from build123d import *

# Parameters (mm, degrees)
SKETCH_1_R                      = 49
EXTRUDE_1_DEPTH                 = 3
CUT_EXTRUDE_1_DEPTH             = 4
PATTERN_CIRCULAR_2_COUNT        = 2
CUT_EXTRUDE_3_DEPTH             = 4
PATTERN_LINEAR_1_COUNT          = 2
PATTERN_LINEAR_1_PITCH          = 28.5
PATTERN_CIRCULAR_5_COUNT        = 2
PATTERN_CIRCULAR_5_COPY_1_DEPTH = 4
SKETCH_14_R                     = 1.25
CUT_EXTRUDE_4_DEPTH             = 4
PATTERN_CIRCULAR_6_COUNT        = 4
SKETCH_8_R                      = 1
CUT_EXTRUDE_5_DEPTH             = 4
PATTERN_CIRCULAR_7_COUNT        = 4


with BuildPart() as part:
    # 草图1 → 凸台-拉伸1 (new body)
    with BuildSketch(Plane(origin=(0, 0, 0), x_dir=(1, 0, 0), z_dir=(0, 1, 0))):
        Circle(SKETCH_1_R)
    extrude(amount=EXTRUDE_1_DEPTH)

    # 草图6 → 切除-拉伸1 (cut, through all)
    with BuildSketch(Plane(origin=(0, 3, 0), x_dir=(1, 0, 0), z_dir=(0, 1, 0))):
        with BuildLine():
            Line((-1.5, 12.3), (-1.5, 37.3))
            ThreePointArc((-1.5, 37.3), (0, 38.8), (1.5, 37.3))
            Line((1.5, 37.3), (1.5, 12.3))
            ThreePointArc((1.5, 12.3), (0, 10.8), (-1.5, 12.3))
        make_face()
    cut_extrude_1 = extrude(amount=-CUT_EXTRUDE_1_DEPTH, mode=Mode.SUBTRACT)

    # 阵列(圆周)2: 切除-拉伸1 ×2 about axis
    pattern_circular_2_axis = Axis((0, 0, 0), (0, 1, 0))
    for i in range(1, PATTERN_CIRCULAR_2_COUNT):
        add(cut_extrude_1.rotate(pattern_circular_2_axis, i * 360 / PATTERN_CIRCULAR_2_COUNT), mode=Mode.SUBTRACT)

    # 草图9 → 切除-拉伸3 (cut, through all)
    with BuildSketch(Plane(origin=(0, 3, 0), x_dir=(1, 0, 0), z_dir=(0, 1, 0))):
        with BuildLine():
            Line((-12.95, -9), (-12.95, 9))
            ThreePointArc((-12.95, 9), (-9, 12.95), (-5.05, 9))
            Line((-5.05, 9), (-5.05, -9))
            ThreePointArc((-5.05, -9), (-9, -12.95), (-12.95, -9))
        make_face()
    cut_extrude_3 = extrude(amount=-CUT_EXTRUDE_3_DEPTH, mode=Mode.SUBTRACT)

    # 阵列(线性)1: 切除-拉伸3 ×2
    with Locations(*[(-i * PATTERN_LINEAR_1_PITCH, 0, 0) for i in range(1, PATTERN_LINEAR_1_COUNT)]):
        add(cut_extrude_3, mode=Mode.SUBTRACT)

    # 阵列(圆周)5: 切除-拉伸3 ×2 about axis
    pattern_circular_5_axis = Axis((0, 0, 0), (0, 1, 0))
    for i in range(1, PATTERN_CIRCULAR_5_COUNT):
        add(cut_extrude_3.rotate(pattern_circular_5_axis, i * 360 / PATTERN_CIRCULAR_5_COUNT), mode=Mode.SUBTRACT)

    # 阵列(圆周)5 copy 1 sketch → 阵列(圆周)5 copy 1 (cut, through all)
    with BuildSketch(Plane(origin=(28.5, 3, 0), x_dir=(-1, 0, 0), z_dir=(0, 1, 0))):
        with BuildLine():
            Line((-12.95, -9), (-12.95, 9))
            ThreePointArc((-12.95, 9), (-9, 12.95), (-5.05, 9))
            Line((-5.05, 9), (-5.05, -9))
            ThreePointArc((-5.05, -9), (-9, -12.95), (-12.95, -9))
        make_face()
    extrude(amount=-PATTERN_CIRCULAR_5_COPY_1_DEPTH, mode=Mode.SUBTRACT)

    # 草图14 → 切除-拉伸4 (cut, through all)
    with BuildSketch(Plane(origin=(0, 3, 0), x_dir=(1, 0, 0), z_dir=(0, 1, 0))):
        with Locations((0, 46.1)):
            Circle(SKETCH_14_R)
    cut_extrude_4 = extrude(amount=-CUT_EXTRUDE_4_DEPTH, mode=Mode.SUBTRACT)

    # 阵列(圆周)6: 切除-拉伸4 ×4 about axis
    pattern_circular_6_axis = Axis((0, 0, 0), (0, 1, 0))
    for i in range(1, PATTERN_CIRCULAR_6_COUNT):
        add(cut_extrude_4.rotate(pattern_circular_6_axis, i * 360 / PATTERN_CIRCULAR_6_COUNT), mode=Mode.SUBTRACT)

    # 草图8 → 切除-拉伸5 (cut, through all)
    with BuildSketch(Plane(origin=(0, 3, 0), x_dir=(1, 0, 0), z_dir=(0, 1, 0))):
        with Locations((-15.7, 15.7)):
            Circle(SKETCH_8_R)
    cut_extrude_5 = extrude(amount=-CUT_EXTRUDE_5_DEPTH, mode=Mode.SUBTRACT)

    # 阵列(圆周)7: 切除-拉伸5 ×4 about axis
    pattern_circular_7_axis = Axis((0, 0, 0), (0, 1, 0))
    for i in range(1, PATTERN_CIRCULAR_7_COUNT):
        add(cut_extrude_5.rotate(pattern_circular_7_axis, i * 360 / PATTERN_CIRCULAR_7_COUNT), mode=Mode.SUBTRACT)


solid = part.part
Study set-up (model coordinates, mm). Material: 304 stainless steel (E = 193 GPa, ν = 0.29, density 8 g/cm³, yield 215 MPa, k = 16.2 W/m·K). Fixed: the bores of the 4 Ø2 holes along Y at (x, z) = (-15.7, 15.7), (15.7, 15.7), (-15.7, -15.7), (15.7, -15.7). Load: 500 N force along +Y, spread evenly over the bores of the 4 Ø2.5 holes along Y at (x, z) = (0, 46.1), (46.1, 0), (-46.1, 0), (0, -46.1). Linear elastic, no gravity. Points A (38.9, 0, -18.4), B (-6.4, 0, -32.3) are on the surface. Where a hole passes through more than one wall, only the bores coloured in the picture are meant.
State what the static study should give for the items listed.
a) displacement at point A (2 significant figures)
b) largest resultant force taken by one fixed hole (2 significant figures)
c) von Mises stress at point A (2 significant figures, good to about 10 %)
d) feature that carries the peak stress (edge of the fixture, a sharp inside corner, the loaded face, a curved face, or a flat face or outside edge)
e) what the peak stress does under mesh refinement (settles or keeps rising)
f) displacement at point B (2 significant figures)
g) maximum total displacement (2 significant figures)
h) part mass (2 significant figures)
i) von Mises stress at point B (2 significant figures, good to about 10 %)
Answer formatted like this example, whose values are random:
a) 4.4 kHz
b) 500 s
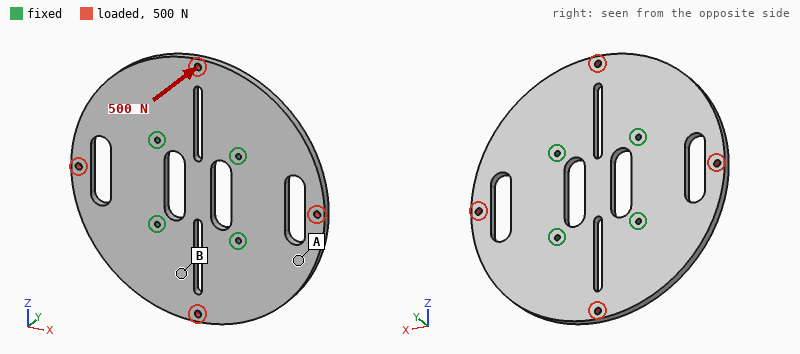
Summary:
a) 33 µm
b) 130 N
c) 37 MPa
d) edge of the fixture
e) keeps rising
f) 18 µm
g) 74 µm
h) 160 g
i) 19 MPa
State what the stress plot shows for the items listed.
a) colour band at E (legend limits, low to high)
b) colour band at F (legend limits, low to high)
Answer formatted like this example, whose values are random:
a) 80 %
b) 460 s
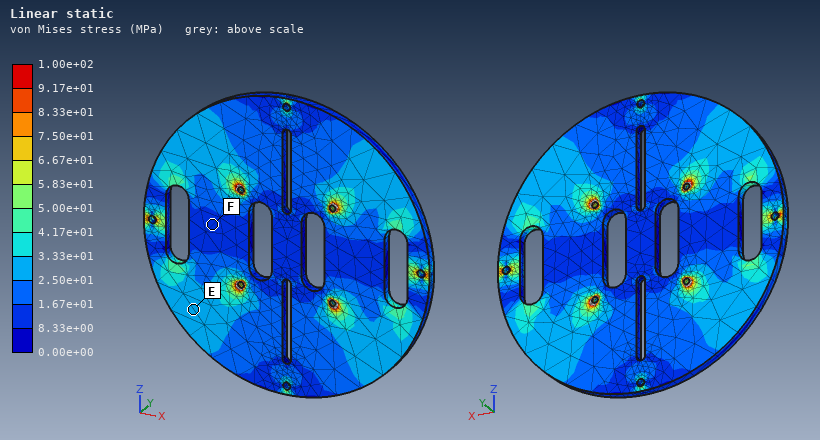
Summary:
a) 2.50e+01 to 3.33e+01 MPa
b) 8.33e+00 to 1.67e+01 MPa
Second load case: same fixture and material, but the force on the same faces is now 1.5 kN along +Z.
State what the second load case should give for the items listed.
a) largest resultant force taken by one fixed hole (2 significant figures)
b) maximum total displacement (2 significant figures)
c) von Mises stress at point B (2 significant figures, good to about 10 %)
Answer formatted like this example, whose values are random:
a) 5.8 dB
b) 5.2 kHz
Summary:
a) 390 N
b) 2.9 µm
c) 6.2 MPa
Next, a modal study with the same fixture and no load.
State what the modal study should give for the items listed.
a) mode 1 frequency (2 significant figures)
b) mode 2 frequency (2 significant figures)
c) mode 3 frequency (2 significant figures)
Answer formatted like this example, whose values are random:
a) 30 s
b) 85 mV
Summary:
a) 2200 Hz
b) 2300 Hz
c) 2300 Hz
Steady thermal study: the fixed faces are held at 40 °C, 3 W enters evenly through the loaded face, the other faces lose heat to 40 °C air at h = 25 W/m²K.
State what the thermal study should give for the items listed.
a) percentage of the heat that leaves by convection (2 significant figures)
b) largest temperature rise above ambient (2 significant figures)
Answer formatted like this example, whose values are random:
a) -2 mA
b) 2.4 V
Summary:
a) 61 %
b) 23 K
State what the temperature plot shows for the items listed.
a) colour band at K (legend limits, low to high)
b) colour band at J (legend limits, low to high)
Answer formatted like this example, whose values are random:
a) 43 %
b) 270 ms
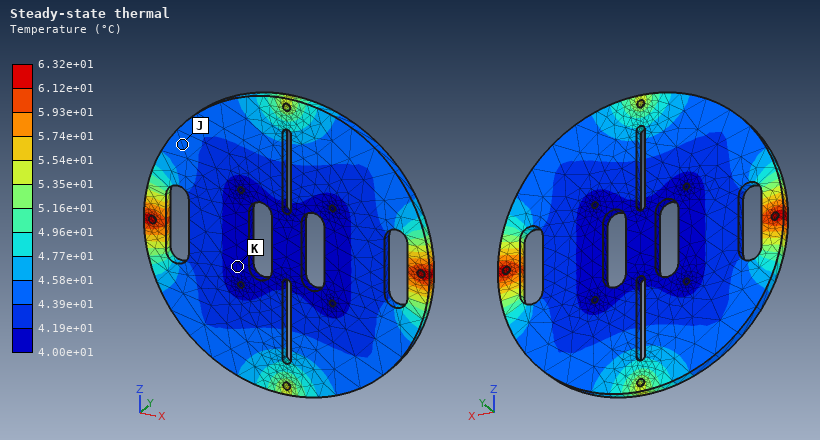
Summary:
a) 4.00e+01 to 4.19e+01 °C
b) 4.39e+01 to 4.58e+01 °C
